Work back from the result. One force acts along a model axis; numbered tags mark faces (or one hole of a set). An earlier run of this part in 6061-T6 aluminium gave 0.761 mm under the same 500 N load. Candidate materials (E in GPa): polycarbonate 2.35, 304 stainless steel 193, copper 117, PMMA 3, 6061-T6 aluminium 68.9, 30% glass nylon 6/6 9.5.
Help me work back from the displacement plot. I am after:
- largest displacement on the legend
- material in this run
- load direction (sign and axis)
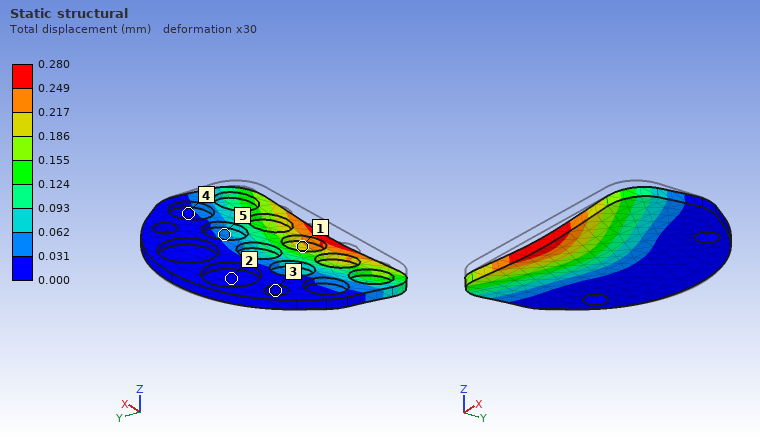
0.280 mm
304 stainless steel
-Z
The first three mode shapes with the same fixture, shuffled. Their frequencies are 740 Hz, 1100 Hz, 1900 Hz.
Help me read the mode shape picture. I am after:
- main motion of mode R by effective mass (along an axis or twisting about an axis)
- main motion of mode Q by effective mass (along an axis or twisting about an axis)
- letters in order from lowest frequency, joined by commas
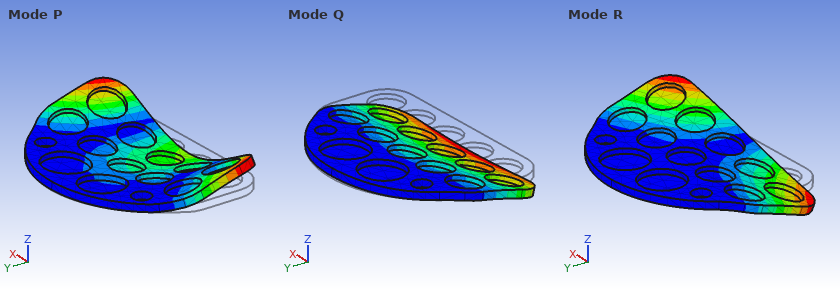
twisting about Y
along Z
Q, R, P
